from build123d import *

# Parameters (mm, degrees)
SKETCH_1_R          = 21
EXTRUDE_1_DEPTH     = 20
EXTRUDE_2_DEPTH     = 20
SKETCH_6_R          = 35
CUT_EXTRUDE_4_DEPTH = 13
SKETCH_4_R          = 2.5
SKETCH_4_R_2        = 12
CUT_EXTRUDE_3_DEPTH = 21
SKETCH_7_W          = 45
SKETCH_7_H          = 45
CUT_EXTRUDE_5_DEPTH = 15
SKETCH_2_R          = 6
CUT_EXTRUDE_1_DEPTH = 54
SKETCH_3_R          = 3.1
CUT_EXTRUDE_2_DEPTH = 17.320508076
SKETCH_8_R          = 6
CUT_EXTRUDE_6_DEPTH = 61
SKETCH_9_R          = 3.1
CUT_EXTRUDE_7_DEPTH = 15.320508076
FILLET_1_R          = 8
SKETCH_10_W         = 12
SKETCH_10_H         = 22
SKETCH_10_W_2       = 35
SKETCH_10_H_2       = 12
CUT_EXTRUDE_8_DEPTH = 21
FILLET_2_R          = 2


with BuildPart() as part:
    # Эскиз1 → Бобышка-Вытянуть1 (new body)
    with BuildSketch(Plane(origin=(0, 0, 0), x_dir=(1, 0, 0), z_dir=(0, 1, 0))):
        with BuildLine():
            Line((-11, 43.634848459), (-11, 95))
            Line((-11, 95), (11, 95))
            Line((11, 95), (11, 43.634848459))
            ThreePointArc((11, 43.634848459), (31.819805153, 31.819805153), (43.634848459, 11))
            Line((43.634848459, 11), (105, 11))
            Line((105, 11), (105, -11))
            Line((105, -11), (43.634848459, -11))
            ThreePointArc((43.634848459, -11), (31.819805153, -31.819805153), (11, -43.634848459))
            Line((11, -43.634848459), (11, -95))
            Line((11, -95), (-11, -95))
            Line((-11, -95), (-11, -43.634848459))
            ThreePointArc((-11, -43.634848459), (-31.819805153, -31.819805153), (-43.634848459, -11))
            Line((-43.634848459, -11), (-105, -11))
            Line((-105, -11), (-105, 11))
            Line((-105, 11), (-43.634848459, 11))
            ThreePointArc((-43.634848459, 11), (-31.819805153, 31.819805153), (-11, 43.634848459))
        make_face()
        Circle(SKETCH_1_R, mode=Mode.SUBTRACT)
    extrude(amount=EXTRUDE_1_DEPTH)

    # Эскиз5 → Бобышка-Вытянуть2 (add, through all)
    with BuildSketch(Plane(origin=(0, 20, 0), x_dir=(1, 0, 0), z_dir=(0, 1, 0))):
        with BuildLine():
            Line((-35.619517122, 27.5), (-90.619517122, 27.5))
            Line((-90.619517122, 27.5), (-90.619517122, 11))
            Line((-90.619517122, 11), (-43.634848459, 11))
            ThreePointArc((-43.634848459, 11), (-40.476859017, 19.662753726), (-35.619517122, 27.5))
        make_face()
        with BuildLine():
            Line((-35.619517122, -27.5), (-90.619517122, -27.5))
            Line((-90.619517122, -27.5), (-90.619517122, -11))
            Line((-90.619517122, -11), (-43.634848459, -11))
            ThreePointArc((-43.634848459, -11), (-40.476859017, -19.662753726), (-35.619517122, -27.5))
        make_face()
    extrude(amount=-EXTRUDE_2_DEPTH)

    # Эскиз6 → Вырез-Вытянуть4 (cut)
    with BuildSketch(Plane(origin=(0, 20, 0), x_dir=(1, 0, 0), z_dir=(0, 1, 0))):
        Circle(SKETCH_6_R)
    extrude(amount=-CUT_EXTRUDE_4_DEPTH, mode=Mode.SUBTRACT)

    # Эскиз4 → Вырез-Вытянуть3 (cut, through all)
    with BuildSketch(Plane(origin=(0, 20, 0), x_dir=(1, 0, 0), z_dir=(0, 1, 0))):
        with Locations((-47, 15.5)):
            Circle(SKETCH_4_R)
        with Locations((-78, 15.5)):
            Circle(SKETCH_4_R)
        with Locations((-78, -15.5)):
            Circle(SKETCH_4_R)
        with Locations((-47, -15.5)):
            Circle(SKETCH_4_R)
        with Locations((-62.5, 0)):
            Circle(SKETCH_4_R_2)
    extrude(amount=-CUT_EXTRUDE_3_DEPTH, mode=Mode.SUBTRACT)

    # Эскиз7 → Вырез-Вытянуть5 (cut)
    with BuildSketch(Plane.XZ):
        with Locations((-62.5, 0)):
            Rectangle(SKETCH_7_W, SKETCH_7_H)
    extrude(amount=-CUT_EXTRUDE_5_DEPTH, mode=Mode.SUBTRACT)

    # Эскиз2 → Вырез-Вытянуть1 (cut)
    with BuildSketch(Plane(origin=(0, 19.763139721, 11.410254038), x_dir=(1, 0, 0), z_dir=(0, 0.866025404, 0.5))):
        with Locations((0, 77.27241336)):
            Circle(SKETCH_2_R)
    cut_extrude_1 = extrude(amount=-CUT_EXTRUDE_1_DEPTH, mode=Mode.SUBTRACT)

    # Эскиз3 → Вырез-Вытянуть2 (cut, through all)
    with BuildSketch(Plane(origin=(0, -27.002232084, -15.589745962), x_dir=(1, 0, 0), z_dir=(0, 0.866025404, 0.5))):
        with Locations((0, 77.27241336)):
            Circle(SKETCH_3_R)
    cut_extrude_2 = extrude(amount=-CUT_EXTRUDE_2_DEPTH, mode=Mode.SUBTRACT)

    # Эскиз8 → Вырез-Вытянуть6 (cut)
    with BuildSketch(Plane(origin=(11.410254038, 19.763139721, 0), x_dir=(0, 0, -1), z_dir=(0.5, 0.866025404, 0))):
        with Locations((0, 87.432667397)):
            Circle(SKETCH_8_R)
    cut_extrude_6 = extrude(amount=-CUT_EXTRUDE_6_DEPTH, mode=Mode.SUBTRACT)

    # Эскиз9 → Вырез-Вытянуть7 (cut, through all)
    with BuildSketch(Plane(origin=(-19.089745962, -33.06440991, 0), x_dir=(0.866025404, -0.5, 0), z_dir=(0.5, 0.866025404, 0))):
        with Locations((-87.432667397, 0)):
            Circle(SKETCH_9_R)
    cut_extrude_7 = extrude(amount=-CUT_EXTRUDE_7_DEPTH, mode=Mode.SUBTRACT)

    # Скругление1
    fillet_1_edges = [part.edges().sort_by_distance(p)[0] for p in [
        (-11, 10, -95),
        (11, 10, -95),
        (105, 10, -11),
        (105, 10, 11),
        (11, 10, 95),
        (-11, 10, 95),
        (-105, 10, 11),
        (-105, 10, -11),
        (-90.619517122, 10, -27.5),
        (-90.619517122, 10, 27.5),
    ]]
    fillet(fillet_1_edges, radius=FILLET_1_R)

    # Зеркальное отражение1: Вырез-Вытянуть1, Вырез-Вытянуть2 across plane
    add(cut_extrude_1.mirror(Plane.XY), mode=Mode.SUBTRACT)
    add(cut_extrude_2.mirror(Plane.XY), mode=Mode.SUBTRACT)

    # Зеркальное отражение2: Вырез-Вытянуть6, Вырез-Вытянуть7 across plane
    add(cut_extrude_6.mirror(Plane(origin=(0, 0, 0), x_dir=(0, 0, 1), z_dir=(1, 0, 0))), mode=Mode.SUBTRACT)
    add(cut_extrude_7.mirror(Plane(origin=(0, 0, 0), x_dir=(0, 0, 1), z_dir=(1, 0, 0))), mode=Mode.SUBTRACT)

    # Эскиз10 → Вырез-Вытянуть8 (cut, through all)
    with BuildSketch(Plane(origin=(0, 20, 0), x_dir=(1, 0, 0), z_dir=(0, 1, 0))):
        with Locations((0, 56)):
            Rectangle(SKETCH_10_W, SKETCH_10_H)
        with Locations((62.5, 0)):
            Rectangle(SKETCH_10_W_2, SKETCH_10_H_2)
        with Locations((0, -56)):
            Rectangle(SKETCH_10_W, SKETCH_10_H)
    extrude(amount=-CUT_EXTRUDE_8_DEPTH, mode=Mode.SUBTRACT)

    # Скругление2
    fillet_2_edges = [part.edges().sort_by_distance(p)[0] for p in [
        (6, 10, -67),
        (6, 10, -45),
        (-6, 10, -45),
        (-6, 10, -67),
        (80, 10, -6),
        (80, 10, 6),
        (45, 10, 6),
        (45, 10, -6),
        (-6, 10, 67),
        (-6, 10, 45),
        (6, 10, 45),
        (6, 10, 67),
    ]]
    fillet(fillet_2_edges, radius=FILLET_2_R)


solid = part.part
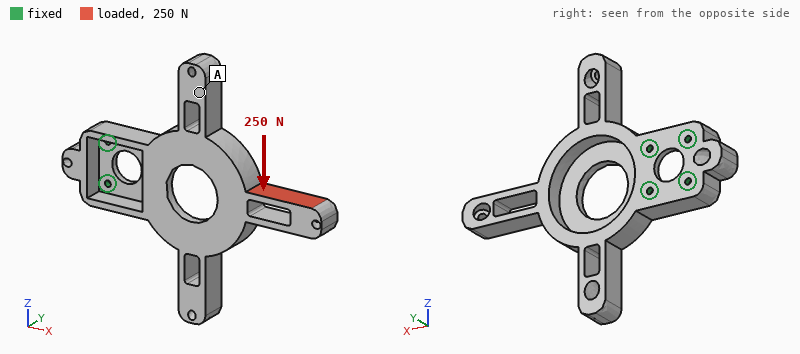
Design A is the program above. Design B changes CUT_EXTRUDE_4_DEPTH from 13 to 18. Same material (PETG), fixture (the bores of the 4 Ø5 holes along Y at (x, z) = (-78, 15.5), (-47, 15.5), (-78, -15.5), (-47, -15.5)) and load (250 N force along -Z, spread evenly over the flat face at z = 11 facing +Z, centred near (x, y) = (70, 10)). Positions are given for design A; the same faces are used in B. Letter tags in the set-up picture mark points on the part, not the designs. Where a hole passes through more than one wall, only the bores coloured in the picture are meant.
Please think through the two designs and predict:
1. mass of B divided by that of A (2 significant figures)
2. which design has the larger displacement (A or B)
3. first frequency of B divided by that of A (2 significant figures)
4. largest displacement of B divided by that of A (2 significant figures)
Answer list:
0.91
B
0.98
1.2
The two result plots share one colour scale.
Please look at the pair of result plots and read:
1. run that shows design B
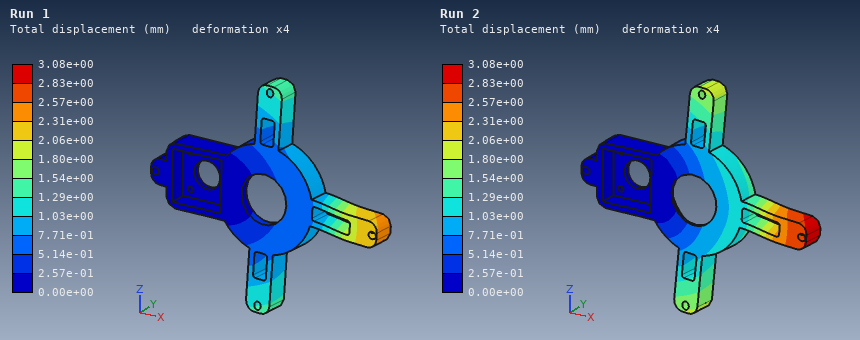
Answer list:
Run 2
